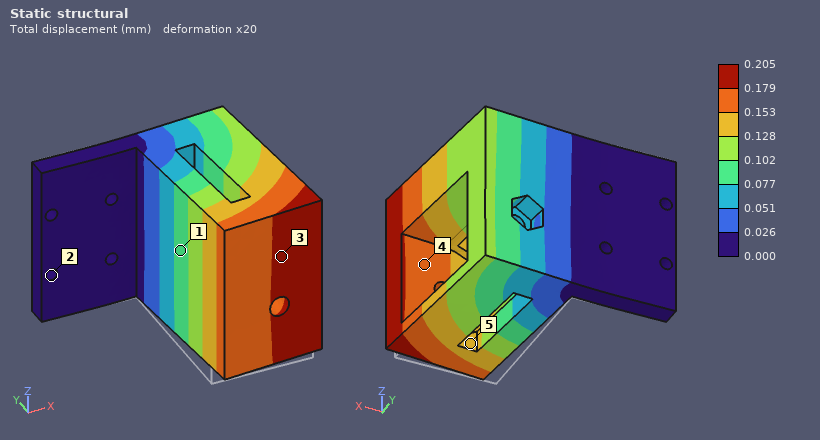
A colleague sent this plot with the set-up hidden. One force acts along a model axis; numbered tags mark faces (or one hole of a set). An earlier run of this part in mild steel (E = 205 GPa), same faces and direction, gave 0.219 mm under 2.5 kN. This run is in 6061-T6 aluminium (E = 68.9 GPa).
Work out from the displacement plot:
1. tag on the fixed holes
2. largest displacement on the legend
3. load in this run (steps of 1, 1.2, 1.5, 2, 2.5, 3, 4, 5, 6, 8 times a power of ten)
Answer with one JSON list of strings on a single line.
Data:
["2", "0.205 mm", "800 N"]
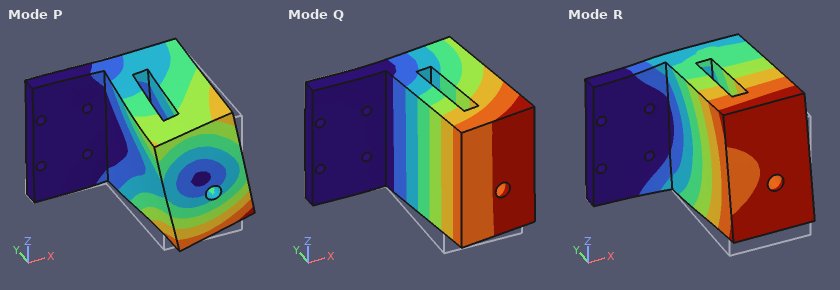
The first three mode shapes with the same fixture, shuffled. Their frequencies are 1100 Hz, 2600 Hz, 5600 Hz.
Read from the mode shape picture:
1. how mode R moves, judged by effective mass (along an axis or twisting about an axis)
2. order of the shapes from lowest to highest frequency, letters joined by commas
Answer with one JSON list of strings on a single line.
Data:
["along Z", "Q, R, P"]
